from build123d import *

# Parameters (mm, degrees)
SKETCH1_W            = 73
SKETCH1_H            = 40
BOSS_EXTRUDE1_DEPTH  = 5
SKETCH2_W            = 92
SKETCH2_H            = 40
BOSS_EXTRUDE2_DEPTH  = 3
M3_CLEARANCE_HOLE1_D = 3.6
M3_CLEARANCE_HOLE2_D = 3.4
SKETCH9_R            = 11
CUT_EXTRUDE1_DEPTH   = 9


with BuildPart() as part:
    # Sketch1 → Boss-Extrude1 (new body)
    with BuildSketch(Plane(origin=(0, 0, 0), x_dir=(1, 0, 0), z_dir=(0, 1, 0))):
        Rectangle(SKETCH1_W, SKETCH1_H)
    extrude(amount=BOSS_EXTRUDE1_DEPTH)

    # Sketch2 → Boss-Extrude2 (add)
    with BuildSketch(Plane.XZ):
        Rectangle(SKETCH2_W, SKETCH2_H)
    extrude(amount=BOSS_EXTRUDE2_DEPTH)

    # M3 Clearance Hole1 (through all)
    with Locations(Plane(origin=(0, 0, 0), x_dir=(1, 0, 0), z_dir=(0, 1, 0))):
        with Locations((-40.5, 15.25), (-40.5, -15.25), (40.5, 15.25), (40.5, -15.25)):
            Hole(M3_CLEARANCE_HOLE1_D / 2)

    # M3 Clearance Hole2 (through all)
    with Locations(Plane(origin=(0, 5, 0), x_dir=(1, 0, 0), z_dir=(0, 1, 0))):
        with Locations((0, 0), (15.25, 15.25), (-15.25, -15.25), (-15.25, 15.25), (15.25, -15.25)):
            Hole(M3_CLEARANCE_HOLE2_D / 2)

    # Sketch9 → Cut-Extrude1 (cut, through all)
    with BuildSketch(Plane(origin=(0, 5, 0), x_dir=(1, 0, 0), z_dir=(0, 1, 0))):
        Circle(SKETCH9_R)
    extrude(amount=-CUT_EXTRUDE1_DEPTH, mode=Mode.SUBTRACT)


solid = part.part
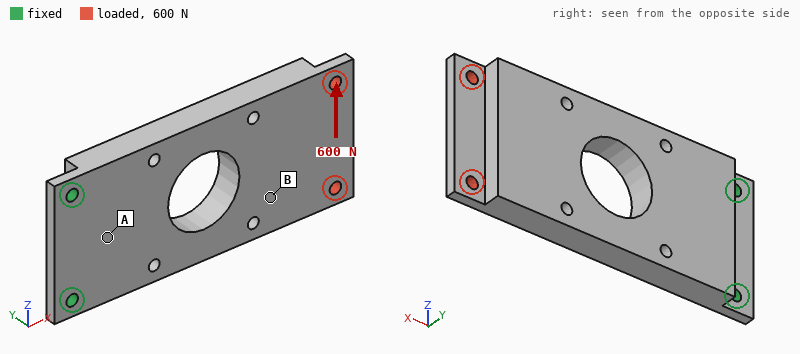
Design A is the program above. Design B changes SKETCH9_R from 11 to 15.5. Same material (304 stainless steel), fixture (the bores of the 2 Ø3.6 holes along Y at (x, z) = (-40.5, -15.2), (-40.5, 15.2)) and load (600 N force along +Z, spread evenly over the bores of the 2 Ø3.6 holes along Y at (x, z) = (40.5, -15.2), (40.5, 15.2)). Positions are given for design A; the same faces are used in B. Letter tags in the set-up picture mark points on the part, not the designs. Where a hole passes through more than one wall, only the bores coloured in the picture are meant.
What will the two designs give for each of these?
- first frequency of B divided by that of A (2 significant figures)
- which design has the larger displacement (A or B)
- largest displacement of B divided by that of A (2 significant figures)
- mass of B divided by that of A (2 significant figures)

1.0
B
1.5
0.86
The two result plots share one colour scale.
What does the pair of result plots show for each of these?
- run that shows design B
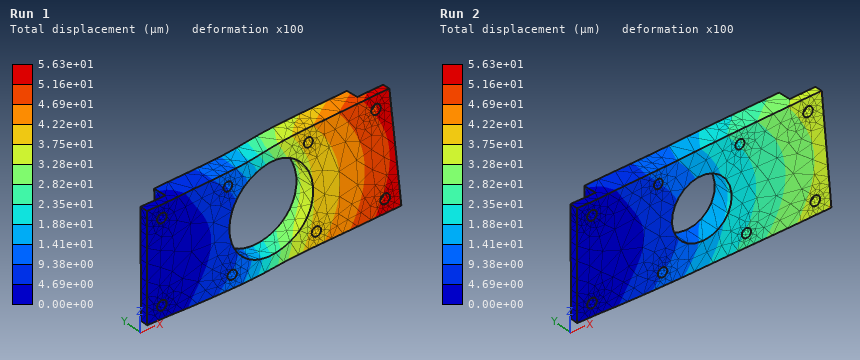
Run 1
